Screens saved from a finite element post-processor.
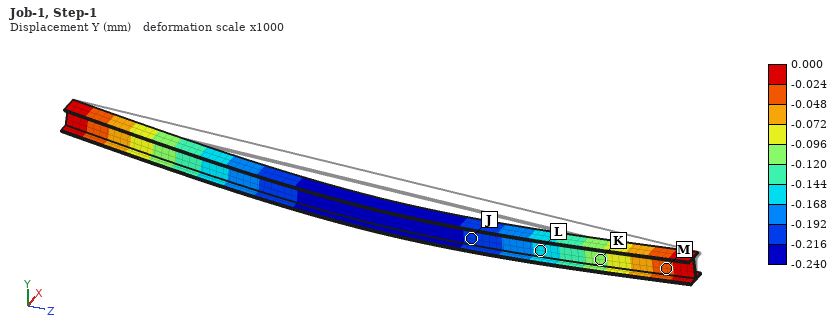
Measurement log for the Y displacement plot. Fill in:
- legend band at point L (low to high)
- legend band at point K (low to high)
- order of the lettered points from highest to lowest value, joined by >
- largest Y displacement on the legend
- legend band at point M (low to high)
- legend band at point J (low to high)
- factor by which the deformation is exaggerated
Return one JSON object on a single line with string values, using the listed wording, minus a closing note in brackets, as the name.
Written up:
{"legend band at point L": "-0.168 to -0.144 mm", "legend band at point K": "-0.120 to -0.096 mm", "order of the lettered points from highest to lowest value, joined by >": "M > K > L > J", "largest Y displacement on the legend": "0.000 mm", "legend band at point M": "-0.048 to -0.024 mm", "legend band at point J": "-0.216 to -0.192 mm", "factor by which the deformation is exaggerated": "1000"}
